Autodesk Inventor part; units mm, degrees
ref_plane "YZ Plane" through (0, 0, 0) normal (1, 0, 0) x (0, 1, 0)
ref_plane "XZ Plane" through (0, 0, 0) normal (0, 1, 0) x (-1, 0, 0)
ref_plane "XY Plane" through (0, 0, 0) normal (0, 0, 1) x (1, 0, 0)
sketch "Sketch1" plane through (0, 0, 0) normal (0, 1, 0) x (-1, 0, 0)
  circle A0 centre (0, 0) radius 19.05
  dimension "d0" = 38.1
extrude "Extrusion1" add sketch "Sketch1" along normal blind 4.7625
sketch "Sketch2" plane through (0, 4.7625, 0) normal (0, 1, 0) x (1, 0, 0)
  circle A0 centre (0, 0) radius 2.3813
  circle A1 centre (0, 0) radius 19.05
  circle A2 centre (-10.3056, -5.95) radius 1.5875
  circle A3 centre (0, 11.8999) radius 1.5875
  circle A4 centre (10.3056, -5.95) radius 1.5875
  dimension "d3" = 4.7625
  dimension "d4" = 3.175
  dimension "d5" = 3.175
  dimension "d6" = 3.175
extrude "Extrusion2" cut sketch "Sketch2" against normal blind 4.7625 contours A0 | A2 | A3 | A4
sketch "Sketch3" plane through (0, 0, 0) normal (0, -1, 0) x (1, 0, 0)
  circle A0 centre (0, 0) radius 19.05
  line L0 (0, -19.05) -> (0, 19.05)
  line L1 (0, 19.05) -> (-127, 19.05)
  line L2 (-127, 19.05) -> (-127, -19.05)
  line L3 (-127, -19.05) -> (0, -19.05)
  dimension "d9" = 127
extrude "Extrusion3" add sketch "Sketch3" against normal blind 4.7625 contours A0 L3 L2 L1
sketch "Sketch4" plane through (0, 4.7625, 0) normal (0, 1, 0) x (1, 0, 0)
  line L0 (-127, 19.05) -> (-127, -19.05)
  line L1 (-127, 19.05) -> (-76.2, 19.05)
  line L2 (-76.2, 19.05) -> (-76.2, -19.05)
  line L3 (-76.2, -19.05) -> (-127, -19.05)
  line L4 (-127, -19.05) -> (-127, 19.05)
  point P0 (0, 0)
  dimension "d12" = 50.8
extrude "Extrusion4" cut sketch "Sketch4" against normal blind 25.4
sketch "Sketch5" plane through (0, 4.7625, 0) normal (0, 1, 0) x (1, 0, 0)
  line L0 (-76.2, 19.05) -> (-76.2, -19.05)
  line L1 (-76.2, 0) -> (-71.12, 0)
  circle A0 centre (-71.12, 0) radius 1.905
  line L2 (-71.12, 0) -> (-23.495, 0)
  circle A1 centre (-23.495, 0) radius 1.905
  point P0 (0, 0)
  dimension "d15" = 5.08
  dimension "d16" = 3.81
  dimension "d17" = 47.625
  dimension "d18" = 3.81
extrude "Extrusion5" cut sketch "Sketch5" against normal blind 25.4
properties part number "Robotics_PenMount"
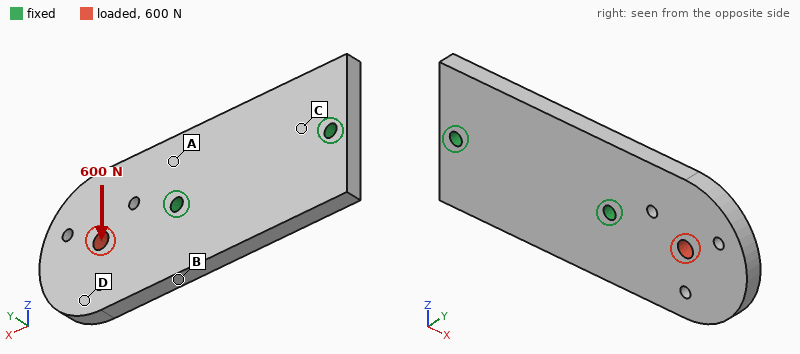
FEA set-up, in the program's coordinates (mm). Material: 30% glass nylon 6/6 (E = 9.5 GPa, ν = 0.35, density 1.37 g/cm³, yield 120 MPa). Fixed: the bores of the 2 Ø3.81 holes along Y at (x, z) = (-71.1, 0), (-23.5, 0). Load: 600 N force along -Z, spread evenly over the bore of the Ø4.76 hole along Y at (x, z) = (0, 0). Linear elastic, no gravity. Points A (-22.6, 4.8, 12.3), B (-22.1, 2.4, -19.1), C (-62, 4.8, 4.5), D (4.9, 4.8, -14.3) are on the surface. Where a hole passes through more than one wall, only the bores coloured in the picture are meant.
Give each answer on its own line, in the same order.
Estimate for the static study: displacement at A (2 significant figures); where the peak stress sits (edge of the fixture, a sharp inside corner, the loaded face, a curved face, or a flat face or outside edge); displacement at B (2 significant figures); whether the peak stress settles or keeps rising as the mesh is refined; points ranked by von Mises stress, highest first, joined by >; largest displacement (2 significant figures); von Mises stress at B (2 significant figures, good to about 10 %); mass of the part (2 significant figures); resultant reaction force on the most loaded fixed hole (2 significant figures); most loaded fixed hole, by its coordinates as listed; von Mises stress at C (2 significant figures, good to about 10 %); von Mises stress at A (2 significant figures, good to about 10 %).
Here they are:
0.022 mm
edge of the fixture
0.037 mm
keeps rising
B > A > C > D
0.13 mm
13 MPa
22 g
870 N
(-23.5, 0)
3.6 MPa
7.5 MPa
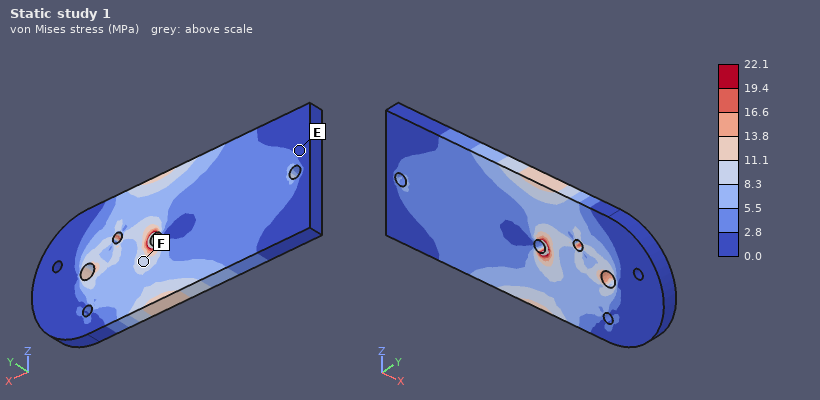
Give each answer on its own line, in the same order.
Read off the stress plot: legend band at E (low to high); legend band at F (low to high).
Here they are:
0.0 to 2.8 MPa
8.3 to 11.1 MPa
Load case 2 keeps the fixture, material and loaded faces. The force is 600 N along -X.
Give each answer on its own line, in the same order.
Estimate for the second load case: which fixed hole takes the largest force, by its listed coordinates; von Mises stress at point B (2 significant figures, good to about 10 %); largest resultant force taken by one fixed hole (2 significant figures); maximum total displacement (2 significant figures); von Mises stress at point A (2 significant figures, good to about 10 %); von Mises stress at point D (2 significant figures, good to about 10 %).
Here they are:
(-23.5, 0)
1.5 MPa
490 N
20 µm
1.9 MPa
1.5 MPa
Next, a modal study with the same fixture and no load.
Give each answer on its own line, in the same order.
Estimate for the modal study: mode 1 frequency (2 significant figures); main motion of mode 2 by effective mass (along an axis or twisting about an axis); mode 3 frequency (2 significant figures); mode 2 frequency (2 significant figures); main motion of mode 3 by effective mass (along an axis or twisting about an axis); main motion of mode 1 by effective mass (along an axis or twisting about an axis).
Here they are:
1200 Hz
twisting about X
3500 Hz
2400 Hz
twisting about X
along Y
